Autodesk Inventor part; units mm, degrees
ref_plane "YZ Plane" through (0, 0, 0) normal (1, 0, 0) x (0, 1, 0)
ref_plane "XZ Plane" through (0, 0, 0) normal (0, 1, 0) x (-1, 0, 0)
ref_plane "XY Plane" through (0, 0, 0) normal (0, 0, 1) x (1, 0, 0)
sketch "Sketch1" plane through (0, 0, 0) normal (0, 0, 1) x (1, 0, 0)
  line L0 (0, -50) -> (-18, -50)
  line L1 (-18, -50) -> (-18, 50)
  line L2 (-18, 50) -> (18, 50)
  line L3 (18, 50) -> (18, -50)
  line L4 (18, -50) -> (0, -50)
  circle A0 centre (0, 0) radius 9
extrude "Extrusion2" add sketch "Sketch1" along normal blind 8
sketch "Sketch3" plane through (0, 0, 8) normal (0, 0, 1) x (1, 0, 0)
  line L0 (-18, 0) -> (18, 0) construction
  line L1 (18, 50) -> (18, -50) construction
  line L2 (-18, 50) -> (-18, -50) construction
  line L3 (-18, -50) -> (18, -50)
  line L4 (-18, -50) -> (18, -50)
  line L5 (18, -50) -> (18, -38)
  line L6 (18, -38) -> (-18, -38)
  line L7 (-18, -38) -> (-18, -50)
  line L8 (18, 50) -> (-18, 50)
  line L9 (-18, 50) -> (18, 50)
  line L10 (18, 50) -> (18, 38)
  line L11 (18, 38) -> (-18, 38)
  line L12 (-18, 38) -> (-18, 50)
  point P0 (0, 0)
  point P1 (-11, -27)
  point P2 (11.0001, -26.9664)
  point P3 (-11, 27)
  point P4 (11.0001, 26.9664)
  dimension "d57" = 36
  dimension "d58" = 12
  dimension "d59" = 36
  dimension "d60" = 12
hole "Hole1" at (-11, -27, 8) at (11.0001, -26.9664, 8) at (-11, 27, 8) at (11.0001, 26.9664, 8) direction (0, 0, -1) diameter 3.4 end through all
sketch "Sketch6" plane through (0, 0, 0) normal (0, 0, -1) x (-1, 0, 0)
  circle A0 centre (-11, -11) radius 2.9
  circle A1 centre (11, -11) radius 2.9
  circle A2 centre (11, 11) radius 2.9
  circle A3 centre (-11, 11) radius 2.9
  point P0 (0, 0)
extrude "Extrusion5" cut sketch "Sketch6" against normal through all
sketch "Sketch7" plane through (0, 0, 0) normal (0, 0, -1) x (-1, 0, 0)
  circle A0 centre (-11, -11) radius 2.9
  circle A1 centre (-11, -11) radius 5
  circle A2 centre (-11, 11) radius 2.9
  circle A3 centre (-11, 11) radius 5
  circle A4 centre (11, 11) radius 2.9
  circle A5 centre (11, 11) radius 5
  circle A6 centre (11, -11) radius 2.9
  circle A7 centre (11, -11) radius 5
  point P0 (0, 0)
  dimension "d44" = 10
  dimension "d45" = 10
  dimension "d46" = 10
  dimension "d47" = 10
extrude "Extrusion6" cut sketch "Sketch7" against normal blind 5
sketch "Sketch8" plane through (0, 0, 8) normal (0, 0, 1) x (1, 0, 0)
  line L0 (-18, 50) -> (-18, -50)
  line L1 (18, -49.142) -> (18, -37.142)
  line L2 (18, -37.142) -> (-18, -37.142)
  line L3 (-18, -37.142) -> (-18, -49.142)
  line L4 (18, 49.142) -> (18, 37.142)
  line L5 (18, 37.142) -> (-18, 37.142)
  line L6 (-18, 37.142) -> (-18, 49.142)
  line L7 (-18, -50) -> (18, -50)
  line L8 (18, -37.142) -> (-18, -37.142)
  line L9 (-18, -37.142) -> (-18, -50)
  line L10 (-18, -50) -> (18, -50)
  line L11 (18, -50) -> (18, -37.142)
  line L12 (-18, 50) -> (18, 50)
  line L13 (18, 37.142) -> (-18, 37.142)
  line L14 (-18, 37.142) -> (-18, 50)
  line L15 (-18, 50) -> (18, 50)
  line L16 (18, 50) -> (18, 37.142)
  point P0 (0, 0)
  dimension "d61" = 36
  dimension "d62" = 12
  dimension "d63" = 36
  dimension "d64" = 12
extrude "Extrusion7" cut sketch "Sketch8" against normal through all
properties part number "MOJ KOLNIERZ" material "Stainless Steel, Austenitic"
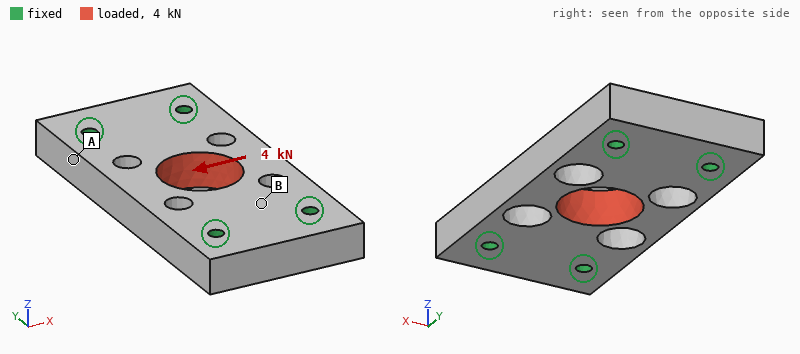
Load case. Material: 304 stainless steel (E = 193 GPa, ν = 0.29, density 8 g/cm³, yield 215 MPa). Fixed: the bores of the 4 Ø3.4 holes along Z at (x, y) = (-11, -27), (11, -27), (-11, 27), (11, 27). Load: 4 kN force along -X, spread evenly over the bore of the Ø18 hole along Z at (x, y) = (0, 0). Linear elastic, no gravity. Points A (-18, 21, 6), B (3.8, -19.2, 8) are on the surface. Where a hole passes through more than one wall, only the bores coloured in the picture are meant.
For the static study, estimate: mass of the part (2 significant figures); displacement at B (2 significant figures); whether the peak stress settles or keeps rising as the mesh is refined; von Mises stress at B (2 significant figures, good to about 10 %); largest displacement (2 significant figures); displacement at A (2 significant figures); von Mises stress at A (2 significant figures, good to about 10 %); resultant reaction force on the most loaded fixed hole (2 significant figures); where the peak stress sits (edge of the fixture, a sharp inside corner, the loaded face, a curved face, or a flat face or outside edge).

140 g
1.0 µm
keeps rising
16 MPa
5.5 µm
1.2 µm
6.1 MPa
1.4 kN
a sharp inside corner
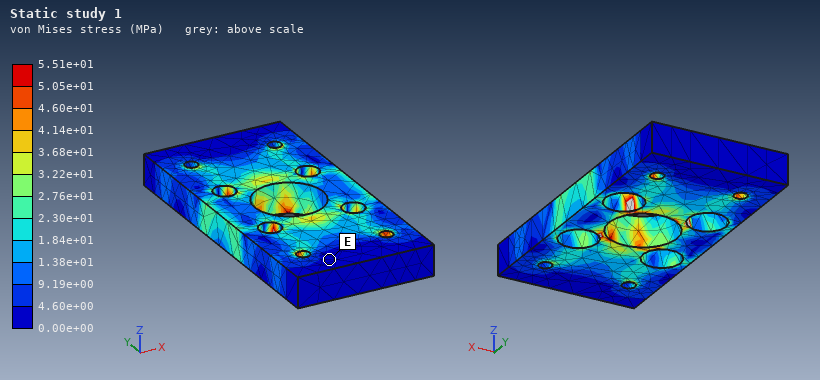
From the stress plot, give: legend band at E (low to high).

0.00e+00 to 4.60e+00 MPa
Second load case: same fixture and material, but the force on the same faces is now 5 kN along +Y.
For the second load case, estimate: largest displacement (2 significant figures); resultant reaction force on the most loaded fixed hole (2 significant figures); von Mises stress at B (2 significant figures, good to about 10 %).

3.8 µm
1.3 kN
12 MPa
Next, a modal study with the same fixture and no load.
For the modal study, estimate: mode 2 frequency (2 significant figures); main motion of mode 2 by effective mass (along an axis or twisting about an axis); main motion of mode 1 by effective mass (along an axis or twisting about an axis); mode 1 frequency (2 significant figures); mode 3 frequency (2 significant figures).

15 kHz
twisting about Y
along Z
12 kHz
24 kHz
